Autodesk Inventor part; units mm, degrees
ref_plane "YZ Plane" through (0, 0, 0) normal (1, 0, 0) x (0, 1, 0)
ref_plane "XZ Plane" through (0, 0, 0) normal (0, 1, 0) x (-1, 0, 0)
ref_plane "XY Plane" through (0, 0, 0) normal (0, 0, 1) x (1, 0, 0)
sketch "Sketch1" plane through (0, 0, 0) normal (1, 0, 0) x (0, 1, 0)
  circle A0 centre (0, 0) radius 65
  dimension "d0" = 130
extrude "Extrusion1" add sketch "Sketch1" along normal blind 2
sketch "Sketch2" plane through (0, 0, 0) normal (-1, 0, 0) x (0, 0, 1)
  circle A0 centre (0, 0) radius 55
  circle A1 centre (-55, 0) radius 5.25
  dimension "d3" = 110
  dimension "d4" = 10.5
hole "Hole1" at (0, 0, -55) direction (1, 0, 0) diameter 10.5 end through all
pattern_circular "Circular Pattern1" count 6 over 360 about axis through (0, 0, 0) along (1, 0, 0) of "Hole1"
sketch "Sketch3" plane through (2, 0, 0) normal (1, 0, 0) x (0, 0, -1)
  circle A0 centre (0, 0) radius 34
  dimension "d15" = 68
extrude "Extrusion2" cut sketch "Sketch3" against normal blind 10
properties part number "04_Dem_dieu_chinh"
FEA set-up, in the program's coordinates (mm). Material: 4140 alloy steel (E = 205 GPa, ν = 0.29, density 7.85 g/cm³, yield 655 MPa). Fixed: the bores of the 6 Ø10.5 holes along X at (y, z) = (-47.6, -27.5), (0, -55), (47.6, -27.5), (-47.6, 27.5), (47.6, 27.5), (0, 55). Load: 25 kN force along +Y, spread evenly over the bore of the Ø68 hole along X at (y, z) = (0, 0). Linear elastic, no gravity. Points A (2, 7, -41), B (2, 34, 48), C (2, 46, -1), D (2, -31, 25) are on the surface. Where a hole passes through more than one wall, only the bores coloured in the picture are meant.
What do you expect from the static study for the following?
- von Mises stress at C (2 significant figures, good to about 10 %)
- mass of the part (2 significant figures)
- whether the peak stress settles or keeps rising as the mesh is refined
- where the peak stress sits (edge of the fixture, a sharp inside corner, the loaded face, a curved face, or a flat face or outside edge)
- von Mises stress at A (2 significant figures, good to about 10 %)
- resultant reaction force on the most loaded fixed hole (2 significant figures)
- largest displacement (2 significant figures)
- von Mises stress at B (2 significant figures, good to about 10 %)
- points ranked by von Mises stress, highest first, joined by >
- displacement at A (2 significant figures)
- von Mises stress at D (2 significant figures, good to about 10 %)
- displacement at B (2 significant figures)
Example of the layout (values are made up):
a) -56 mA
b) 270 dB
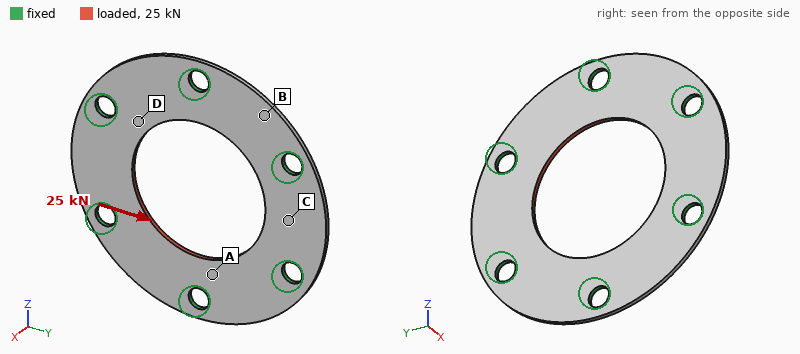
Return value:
a) 32 MPa
b) 140 g
c) keeps rising
d) edge of the fixture
e) 57 MPa
f) 4.8 kN
g) 13 µm
h) 16 MPa
i) D > A > C > B
j) 7.0 µm
k) 98 MPa
l) 5.1 µm
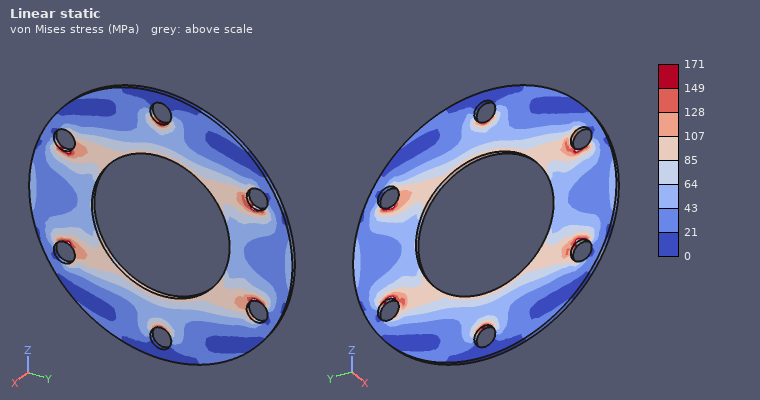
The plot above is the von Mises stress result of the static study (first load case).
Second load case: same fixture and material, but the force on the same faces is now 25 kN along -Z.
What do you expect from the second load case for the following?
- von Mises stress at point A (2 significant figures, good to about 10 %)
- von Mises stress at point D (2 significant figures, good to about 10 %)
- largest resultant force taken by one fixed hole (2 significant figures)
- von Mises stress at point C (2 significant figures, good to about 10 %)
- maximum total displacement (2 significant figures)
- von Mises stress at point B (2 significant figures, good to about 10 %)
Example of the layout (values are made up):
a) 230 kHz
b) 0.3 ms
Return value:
a) 91 MPa
b) 45 MPa
c) 5.3 kN
d) 46 MPa
e) 13 µm
f) 32 MPa
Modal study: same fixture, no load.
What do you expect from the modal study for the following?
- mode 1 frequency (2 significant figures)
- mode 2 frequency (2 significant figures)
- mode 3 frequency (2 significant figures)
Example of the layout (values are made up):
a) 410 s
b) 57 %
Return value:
a) 4000 Hz
b) 4100 Hz
c) 4100 Hz
